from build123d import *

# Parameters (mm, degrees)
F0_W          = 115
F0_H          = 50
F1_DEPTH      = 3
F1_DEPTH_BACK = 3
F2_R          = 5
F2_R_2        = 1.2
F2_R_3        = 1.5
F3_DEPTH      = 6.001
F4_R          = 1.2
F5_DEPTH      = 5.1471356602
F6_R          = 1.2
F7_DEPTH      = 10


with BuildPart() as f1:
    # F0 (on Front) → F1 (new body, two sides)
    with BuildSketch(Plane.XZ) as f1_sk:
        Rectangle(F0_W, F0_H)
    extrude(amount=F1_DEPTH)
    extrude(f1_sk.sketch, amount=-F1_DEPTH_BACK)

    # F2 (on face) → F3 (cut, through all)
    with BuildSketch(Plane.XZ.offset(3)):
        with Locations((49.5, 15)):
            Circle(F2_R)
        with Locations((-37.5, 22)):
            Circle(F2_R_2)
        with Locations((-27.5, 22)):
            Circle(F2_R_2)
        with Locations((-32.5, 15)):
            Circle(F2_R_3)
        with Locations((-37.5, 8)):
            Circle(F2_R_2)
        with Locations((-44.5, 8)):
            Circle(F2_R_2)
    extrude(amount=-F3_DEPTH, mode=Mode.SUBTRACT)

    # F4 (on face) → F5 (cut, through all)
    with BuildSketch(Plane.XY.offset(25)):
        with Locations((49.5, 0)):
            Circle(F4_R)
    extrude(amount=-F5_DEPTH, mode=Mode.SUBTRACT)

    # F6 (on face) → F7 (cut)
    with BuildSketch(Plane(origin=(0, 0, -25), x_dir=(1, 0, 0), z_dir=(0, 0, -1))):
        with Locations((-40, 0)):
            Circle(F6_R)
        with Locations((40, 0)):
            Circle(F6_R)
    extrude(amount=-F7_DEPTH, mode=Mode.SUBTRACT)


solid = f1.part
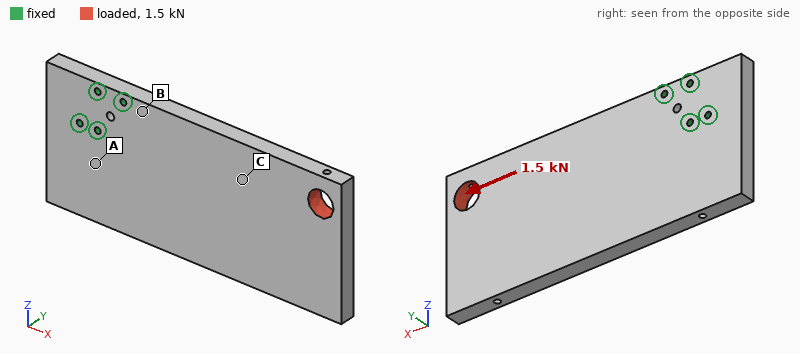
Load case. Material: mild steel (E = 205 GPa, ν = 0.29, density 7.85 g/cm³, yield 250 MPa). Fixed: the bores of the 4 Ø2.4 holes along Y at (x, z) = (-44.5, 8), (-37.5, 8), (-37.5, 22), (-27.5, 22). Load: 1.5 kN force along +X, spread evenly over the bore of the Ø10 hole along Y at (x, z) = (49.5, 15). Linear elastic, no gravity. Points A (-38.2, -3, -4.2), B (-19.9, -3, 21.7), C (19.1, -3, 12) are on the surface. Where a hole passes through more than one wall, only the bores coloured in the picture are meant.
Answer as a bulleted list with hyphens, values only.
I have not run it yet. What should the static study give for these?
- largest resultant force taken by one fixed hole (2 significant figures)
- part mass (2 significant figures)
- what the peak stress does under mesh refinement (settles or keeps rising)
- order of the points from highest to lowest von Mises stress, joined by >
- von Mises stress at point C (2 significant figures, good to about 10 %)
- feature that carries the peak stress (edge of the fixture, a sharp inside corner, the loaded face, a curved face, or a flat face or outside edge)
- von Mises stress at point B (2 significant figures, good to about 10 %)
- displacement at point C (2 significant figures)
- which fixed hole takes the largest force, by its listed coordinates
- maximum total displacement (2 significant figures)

- 700 N
- 270 g
- keeps rising
- B > C > A
- 9.1 MPa
- a sharp inside corner
- 15 MPa
- 2.7 µm
- (-27.5, 22)
- 7.9 µm
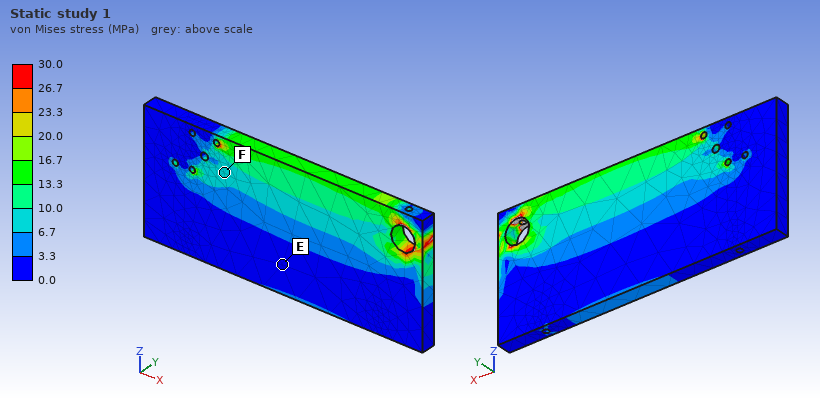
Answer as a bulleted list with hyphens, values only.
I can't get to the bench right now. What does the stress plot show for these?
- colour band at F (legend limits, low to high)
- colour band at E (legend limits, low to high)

- 6.7 to 10.0 MPa
- 0.0 to 3.3 MPa
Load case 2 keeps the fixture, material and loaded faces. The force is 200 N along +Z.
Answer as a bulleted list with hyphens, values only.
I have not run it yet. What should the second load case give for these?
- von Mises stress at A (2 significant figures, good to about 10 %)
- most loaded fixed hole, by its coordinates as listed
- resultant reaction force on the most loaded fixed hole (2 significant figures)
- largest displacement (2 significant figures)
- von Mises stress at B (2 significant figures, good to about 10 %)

- 4.2 MPa
- (-27.5, 22)
- 650 N
- 8.9 µm
- 8.7 MPa
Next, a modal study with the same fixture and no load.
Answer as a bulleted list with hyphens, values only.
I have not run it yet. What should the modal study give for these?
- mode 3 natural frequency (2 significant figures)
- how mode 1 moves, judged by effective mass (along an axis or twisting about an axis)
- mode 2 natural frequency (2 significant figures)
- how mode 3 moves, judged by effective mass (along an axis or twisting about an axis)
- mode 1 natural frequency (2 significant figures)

- 2800 Hz
- along Y
- 2000 Hz
- along Z
- 560 Hz
